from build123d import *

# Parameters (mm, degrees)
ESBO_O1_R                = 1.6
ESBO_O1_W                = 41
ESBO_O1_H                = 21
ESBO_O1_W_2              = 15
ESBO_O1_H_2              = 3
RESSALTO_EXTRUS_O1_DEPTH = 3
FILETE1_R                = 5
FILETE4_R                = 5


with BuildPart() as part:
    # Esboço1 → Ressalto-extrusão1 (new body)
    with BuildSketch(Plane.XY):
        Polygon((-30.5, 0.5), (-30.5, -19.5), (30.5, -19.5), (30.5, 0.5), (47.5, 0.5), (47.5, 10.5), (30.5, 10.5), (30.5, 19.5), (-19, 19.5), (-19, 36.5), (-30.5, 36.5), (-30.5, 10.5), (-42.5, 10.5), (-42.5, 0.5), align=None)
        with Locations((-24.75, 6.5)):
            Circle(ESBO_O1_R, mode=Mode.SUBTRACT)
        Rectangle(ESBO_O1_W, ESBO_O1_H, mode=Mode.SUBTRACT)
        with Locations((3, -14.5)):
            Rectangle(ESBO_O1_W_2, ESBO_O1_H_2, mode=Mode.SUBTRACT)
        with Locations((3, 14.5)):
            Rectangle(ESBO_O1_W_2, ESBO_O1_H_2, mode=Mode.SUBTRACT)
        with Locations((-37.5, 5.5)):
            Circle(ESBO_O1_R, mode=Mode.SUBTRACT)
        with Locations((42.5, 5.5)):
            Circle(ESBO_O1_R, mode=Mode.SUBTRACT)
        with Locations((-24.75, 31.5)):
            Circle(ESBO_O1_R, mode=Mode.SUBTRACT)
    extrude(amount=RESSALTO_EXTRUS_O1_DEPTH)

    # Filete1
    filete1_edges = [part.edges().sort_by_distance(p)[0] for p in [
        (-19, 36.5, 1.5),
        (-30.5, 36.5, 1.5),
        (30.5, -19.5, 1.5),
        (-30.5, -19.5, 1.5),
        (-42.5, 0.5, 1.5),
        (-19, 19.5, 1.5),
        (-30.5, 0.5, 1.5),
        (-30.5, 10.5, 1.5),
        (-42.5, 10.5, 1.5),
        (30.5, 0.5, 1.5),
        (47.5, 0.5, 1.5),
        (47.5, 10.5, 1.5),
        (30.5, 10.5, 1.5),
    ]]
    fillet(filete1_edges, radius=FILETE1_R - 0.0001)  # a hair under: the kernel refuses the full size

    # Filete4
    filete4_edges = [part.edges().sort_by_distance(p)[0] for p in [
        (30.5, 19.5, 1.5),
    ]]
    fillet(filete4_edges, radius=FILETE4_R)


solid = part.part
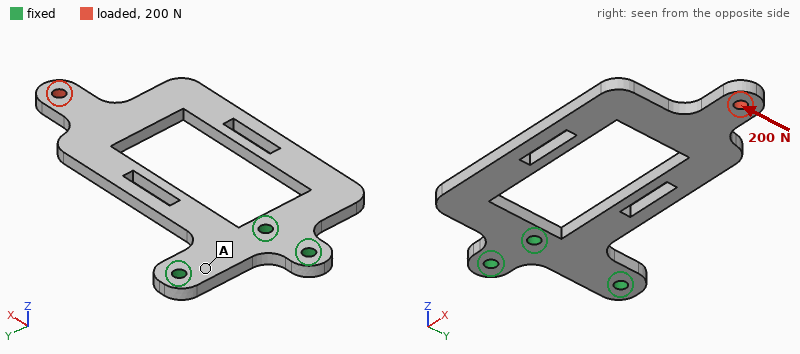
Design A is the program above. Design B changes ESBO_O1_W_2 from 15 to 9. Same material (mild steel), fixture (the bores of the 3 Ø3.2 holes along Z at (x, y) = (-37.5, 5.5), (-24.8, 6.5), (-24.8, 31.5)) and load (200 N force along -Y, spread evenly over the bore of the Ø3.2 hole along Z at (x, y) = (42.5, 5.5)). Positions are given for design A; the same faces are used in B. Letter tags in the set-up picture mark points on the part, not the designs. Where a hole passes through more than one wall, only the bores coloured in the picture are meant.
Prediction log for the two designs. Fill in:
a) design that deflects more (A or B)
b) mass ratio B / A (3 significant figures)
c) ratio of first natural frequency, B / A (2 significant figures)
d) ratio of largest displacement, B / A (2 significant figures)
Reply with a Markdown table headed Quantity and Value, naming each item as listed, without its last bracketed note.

| Quantity | Value |
|---|---|
| design that deflects more | A |
| mass ratio B / A | 1.02 |
| ratio of first natural frequency, B / A | 1.0 |
| ratio of largest displacement, B / A | 0.87 |
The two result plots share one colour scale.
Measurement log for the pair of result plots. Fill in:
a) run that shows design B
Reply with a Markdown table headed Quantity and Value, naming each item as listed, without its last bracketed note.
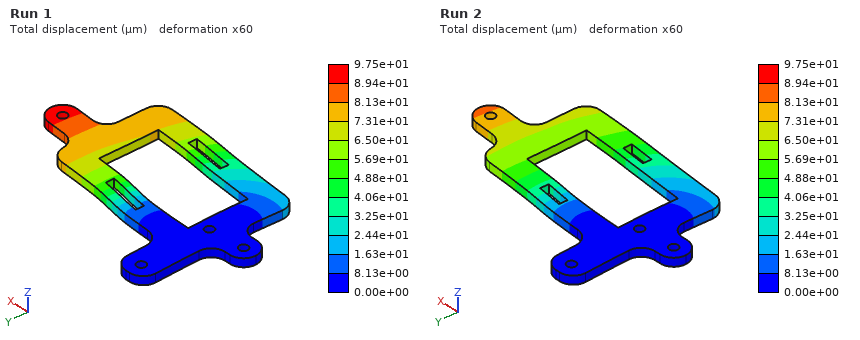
| Quantity | Value |
|---|---|
| run that shows design B | Run 2 |
